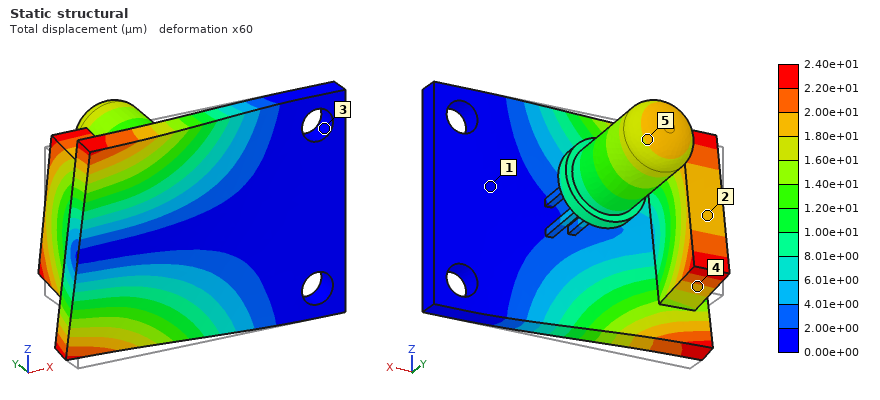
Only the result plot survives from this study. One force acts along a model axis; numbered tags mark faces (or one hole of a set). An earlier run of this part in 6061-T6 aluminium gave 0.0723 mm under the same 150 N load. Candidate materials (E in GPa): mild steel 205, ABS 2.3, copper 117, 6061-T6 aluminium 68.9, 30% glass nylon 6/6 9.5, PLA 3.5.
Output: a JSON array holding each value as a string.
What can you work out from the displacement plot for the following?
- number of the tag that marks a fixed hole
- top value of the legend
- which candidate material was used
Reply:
["3", "2.40e+01 µm", "mild steel"]
